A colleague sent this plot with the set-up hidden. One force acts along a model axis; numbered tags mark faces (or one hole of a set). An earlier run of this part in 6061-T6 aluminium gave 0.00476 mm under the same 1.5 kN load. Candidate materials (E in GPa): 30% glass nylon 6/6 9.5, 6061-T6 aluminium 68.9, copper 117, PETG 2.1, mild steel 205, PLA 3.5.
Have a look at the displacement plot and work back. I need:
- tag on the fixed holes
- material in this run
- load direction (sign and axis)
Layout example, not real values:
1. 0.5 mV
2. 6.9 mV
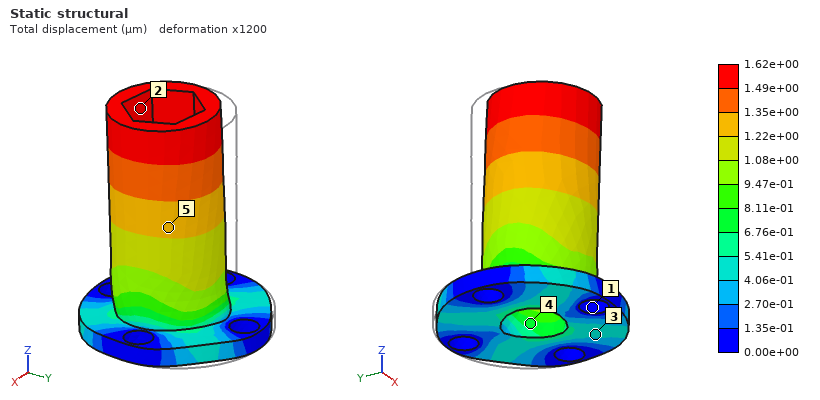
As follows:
1. 1
2. mild steel
3. -Y
